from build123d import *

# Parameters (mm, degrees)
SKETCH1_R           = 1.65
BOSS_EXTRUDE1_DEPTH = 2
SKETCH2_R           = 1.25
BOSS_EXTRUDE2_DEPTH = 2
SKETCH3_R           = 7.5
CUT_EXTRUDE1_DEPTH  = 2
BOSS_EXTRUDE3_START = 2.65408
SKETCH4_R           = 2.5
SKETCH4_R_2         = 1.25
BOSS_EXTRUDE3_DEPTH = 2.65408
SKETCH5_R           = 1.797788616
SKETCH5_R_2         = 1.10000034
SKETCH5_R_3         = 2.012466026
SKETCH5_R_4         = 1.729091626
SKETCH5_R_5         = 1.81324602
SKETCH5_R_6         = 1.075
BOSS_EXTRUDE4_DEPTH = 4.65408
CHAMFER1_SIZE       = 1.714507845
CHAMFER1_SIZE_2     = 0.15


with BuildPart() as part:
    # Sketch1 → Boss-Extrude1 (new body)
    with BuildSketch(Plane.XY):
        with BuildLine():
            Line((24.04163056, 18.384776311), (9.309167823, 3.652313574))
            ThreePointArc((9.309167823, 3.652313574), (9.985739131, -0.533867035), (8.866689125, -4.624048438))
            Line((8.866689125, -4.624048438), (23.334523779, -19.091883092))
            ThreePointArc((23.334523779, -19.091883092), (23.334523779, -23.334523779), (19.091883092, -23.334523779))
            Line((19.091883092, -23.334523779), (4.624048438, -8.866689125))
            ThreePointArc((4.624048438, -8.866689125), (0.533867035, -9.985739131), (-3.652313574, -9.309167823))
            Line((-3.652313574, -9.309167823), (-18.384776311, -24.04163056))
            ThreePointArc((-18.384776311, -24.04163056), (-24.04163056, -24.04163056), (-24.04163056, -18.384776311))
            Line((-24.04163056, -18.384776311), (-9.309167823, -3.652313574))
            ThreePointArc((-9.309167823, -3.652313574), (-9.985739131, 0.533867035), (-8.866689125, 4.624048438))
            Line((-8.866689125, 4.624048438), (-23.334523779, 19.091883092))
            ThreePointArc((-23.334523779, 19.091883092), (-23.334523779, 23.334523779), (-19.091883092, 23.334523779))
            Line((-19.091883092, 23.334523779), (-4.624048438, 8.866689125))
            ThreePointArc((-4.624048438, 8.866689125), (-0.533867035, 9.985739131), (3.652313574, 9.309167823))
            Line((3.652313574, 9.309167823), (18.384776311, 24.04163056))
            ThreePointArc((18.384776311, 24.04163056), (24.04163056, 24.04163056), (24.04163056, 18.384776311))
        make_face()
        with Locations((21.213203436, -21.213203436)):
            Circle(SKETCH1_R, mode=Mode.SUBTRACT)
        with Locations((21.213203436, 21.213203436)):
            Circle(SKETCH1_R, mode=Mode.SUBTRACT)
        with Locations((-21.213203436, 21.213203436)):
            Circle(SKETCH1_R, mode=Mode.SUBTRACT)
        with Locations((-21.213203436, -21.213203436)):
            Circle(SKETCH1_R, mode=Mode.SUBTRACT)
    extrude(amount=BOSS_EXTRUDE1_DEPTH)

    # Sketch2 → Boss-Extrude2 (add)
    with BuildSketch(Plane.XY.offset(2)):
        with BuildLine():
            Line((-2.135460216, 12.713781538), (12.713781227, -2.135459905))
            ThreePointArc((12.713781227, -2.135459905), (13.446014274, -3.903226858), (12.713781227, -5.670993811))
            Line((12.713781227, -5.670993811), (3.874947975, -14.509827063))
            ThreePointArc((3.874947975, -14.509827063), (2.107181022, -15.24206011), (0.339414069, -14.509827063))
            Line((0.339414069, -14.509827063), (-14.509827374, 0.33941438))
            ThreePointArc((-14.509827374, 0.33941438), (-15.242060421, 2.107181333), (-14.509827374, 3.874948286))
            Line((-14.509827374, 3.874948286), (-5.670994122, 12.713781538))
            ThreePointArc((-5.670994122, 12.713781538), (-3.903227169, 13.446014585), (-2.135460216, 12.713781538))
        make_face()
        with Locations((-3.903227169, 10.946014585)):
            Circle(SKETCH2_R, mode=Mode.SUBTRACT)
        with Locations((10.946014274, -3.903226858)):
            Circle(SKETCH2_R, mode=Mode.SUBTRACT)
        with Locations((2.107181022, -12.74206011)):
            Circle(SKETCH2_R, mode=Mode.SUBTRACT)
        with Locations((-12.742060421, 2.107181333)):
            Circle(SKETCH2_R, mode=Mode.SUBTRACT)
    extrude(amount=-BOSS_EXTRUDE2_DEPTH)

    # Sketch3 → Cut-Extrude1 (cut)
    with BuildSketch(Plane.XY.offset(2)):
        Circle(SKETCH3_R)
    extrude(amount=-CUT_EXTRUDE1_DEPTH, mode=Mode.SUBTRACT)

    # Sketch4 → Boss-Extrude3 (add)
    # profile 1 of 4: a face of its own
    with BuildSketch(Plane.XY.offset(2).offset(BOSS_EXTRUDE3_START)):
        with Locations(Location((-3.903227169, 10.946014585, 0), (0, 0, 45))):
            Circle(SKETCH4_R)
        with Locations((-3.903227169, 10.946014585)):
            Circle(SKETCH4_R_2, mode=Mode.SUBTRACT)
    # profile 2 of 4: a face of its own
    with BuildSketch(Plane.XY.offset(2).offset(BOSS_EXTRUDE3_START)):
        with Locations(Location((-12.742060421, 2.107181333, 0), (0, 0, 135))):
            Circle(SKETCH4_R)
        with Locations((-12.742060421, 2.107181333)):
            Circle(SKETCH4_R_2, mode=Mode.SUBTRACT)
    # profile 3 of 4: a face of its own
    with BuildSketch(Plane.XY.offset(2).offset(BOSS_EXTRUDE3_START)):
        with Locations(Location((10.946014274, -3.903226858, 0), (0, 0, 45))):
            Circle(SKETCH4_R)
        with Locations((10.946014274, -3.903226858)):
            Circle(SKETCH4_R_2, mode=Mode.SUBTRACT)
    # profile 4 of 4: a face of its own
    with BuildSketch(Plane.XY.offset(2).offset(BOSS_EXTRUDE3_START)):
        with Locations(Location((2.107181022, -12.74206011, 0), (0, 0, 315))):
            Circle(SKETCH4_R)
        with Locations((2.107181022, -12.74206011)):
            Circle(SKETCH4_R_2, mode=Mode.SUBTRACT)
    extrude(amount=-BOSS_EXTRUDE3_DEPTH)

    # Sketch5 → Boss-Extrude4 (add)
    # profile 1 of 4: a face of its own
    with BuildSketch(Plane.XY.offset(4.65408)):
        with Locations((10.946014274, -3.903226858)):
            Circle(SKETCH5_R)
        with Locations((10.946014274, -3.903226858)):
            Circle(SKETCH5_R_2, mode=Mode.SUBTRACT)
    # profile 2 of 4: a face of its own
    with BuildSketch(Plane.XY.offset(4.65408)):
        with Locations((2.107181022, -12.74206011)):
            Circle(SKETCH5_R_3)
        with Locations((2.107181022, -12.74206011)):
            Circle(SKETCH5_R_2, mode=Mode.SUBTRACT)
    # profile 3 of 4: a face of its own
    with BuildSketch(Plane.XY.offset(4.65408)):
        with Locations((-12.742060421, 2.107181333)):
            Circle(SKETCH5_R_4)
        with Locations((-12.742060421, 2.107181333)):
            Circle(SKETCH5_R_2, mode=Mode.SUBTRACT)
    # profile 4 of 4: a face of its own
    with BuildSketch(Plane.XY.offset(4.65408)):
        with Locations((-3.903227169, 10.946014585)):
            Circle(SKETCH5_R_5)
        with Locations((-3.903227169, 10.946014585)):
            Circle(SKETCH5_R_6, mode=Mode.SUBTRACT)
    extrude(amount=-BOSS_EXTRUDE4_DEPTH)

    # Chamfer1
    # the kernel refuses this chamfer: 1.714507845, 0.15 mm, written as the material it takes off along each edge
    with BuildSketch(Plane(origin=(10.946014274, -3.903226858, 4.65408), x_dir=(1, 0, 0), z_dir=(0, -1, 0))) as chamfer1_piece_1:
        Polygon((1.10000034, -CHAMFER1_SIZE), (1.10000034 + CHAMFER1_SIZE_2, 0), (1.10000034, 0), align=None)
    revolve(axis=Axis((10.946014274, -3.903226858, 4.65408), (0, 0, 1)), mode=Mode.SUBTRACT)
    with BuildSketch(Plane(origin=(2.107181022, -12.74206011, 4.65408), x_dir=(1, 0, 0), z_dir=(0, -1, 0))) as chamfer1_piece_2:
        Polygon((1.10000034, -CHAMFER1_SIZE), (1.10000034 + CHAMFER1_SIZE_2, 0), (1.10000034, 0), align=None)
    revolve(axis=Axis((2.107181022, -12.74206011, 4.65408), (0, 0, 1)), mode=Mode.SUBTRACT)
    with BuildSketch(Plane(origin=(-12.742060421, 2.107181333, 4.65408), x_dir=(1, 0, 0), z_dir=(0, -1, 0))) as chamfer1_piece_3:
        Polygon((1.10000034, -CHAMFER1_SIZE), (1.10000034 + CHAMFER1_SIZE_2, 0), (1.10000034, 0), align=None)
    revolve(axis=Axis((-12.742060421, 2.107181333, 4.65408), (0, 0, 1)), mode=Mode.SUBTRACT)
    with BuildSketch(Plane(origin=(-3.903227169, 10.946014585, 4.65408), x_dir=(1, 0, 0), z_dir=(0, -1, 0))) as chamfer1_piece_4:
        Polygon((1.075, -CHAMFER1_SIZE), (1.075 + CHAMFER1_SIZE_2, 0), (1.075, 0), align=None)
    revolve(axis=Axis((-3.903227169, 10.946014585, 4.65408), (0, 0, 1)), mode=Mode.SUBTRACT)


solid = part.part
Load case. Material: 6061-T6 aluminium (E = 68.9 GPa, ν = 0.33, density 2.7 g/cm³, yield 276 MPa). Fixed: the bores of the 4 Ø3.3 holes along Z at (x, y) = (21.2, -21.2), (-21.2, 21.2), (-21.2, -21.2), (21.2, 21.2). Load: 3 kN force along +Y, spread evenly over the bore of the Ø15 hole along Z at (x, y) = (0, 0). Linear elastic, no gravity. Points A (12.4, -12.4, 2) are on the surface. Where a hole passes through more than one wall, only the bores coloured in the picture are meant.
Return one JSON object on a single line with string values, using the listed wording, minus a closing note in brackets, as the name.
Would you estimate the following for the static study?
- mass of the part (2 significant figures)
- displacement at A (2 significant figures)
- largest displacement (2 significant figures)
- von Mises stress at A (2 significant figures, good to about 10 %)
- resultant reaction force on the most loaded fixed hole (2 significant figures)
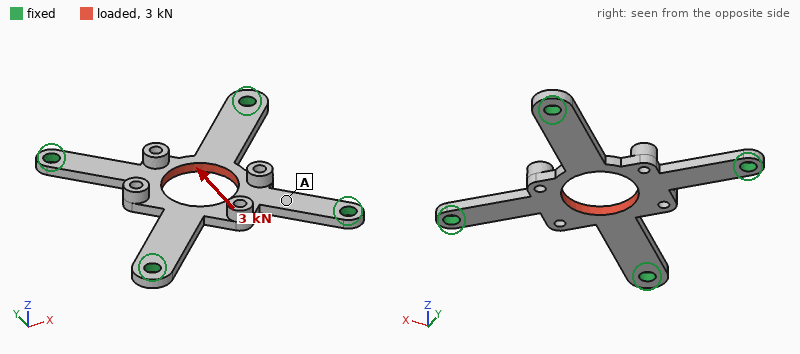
{"mass of the part": "5.0 g", "displacement at A": "24 µm", "largest displacement": "60 µm", "von Mises stress at A": "83 MPa", "resultant reaction force on the most loaded fixed hole": "1.0 kN"}
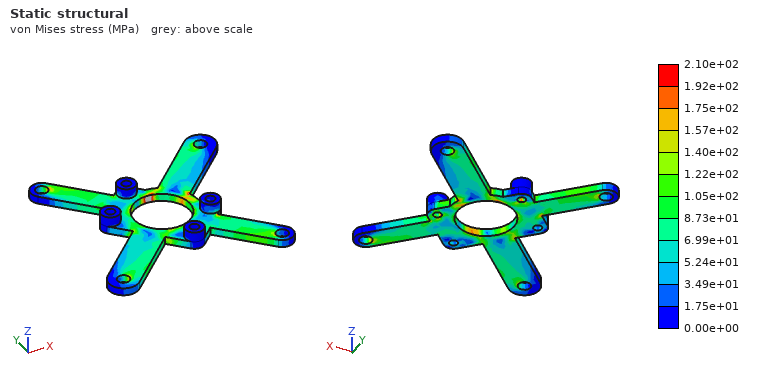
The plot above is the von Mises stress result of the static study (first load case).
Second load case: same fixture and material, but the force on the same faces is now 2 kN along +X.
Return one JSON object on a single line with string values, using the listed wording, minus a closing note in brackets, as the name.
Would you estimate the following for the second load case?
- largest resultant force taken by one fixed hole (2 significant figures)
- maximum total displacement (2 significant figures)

{"largest resultant force taken by one fixed hole": "700 N", "maximum total displacement": "40 µm"}
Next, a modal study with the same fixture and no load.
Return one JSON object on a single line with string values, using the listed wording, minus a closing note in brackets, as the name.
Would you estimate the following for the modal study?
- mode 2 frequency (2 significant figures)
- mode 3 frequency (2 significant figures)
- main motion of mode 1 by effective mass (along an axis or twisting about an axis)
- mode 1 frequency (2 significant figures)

{"mode 2 frequency": "6700 Hz", "mode 3 frequency": "6800 Hz", "main motion of mode 1 by effective mass": "along Z", "mode 1 frequency": "3400 Hz"}
